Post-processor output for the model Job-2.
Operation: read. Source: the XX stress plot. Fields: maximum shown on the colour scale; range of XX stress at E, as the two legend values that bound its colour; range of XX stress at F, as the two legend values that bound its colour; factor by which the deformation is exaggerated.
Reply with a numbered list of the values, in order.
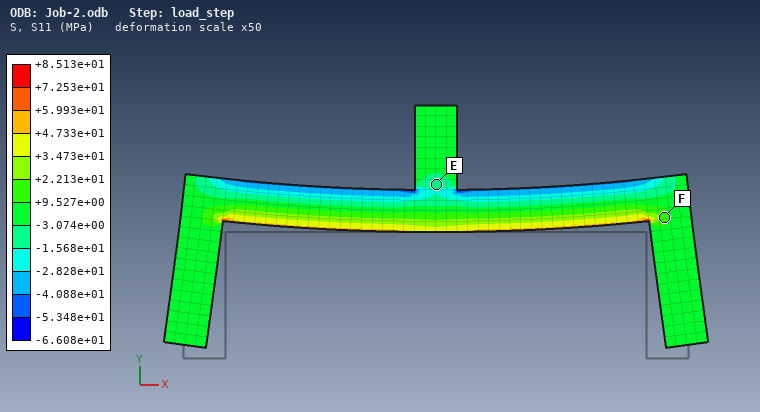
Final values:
1. +8.513e+01 MPa
2. -1.568e+01 to -3.074e+00 MPa
3. +9.527e+00 to +2.213e+01 MPa
4. 50
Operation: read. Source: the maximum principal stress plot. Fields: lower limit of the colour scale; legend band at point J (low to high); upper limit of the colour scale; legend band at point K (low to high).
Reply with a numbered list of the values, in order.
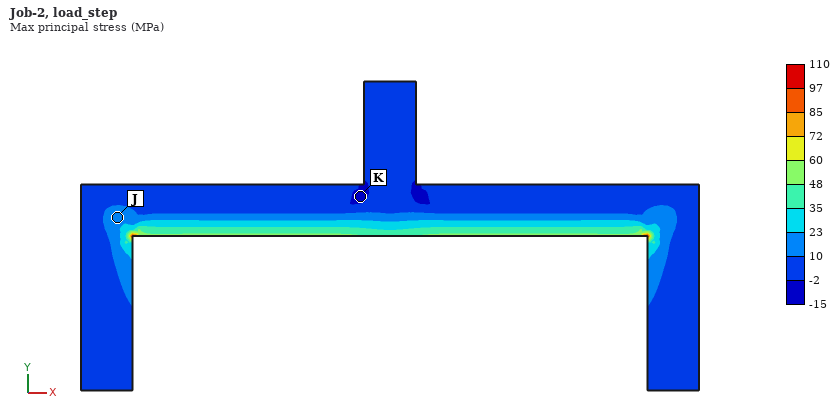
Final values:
1. -15 MPa
2. 10 to 23 MPa
3. 110 MPa
4. -15 to -2 MPa
